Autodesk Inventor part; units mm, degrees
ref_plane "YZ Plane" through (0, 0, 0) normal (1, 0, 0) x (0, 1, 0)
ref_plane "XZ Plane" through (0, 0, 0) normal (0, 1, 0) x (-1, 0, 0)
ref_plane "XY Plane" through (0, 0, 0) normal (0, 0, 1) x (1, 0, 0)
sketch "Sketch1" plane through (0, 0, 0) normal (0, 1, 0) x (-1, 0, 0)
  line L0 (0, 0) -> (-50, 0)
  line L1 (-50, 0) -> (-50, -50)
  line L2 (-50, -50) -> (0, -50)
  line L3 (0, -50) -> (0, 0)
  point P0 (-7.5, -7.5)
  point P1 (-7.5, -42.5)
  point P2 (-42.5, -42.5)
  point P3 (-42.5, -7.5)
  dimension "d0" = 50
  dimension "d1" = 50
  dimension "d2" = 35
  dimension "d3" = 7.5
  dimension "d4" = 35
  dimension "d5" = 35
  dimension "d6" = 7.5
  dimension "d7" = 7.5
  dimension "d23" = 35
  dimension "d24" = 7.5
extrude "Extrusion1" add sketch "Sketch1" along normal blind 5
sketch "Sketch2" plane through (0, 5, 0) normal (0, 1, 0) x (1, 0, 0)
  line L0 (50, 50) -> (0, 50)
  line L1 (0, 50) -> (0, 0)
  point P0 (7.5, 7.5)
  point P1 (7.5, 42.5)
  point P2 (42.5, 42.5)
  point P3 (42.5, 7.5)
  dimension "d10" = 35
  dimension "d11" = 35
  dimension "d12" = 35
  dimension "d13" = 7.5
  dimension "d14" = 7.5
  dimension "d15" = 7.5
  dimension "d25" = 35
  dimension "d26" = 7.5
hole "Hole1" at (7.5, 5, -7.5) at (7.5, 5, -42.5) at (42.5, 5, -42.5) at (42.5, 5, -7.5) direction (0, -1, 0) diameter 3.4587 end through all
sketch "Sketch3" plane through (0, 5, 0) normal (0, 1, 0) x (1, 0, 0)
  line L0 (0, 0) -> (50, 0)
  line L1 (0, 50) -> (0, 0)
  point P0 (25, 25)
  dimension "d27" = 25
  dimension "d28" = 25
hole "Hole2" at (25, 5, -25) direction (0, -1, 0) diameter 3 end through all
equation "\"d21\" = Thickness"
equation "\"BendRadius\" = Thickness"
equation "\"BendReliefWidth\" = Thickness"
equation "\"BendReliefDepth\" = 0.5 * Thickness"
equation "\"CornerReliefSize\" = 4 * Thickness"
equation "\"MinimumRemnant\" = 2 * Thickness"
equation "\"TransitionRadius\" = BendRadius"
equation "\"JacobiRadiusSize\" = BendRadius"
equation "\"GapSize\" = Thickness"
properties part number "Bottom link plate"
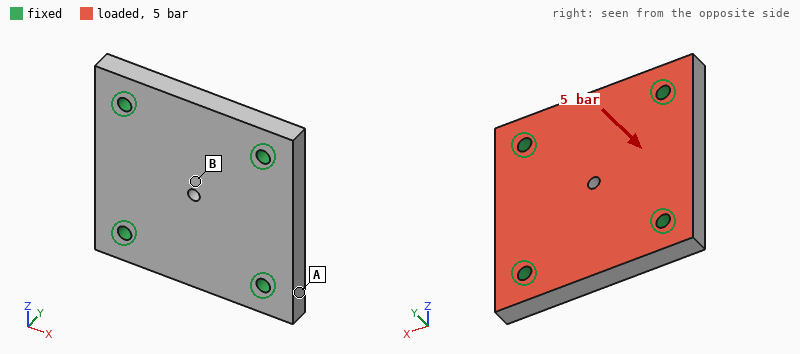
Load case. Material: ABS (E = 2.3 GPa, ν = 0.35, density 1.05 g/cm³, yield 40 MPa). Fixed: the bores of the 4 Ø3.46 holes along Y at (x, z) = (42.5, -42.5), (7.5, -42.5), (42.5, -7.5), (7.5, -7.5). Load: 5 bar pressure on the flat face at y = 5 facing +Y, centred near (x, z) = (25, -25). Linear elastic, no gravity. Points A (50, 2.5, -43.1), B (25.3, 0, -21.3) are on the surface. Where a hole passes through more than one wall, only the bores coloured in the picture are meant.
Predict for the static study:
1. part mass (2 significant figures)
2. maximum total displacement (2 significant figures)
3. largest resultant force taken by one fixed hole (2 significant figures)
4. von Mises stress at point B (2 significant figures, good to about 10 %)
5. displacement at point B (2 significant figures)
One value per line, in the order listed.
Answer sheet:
13 g
0.22 mm
310 N
7.3 MPa
0.21 mm
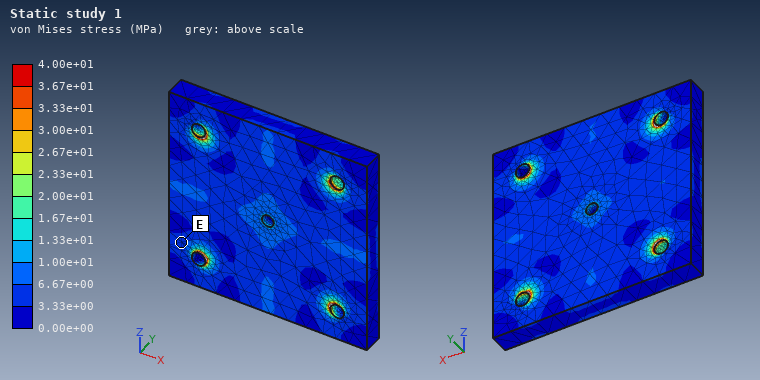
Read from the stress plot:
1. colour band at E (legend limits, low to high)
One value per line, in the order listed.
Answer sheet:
3.33e+00 to 6.67e+00 MPa
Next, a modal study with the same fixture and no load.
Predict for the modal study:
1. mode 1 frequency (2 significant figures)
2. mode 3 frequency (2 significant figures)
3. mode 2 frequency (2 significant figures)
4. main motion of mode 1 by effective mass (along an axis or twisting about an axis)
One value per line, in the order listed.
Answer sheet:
4000 Hz
5800 Hz
5700 Hz
along Y
